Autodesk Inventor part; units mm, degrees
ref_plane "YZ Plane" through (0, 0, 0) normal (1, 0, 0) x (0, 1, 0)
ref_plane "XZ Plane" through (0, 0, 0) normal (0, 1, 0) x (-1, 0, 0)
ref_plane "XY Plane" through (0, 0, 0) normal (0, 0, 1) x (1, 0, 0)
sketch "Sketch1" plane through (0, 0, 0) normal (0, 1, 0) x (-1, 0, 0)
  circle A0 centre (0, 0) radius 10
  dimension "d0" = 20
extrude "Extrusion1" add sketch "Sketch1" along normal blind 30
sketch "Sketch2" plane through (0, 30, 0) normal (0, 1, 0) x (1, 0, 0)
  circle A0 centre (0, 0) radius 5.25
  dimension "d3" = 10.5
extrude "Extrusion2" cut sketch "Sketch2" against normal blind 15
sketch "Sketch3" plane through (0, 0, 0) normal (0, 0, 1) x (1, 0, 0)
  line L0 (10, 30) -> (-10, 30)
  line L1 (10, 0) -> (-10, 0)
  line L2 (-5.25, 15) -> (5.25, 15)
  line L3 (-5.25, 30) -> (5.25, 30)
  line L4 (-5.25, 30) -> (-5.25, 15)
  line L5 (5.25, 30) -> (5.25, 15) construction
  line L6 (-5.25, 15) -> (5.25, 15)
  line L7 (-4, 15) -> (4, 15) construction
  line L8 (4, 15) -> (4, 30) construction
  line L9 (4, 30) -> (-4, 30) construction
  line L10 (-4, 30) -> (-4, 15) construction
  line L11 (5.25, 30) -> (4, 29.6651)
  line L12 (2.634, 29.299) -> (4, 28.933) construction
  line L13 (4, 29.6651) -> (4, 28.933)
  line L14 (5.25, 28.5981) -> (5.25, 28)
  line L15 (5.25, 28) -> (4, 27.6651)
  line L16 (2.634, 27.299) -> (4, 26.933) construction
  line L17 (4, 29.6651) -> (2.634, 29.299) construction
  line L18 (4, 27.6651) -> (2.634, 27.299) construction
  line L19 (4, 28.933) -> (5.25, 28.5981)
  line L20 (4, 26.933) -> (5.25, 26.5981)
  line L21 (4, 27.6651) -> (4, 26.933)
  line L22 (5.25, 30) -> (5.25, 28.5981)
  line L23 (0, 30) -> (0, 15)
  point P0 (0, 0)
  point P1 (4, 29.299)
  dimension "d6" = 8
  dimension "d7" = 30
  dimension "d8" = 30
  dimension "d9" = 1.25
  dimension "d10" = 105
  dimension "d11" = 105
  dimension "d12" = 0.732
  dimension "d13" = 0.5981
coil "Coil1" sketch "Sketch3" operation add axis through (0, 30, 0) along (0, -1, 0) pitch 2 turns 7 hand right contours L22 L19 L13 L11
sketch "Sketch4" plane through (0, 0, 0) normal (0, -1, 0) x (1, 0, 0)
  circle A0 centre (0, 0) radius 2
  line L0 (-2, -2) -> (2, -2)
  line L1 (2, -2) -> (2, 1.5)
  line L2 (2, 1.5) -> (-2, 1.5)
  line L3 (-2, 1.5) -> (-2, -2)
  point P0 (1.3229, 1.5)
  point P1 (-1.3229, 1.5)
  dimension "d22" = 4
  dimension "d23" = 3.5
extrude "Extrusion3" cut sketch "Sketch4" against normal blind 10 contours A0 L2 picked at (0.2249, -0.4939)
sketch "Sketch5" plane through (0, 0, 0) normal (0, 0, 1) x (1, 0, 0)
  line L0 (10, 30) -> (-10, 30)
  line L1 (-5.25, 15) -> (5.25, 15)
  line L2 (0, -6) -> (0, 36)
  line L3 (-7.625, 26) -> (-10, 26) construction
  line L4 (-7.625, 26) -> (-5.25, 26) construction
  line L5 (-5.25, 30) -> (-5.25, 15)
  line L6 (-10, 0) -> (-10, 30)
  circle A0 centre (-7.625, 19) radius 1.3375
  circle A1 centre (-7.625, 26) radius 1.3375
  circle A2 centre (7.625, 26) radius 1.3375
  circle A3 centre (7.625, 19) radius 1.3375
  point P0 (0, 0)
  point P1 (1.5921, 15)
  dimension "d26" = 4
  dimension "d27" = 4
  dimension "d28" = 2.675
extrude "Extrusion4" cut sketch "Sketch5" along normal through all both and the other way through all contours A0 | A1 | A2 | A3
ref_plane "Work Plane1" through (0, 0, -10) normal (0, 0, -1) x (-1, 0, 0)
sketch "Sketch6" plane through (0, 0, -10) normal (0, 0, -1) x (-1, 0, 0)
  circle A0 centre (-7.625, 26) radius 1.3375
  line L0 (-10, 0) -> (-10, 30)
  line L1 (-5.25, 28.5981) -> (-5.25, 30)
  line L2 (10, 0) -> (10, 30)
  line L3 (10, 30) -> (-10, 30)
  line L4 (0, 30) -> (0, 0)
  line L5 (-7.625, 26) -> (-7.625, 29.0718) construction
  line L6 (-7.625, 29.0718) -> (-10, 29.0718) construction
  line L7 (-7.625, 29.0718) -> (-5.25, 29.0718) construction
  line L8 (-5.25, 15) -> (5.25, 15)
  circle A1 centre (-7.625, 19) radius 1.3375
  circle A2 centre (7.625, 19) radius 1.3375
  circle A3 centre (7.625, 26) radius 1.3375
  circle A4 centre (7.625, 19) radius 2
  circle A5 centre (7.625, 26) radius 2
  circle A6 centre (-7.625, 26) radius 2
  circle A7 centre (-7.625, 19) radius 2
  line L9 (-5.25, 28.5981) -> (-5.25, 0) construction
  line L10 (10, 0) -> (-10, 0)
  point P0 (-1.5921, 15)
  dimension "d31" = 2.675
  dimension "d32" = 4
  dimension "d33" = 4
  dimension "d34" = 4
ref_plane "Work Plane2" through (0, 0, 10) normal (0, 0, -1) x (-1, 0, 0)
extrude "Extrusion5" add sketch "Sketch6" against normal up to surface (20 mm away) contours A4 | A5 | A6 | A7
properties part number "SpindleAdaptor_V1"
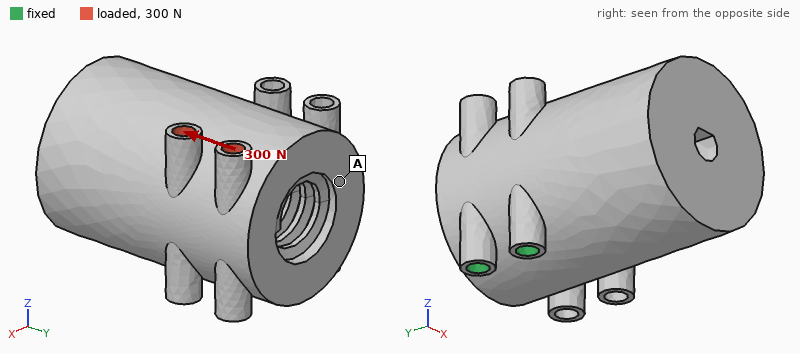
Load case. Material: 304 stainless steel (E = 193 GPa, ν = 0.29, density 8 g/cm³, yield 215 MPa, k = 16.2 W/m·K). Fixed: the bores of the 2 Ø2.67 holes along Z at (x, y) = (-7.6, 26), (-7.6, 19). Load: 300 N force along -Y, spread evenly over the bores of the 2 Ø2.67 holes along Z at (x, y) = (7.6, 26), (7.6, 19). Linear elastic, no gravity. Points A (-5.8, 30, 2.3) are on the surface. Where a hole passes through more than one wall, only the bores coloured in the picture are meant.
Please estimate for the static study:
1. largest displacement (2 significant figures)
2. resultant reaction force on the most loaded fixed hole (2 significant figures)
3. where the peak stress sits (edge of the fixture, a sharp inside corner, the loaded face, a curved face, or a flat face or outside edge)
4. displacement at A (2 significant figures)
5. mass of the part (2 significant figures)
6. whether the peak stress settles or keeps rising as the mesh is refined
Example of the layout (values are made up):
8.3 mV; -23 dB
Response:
11 µm; 830 N; edge of the fixture; 3.8 µm; 66 g; keeps rising
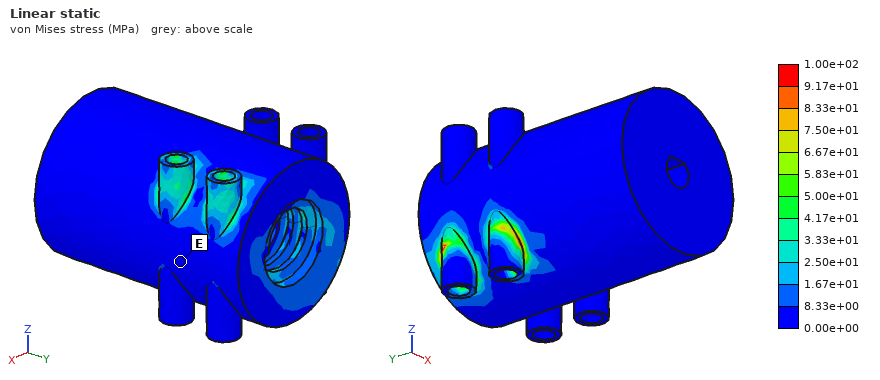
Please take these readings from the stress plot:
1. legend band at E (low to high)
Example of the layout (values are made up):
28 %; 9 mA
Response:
0.00e+00 to 8.33e+00 MPa
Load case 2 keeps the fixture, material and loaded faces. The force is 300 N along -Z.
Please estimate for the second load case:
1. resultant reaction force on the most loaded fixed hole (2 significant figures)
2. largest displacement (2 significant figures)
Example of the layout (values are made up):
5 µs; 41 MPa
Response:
160 N; 25 µm
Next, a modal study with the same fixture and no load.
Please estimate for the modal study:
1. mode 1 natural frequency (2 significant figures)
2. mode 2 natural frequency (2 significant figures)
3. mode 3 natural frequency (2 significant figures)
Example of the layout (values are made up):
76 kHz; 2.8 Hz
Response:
3100 Hz; 5000 Hz; 7200 Hz
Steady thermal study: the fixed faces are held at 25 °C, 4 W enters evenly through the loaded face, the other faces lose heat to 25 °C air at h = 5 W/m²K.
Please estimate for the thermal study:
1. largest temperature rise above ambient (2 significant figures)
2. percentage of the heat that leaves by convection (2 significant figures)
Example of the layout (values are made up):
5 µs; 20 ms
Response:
76 K; 13 %
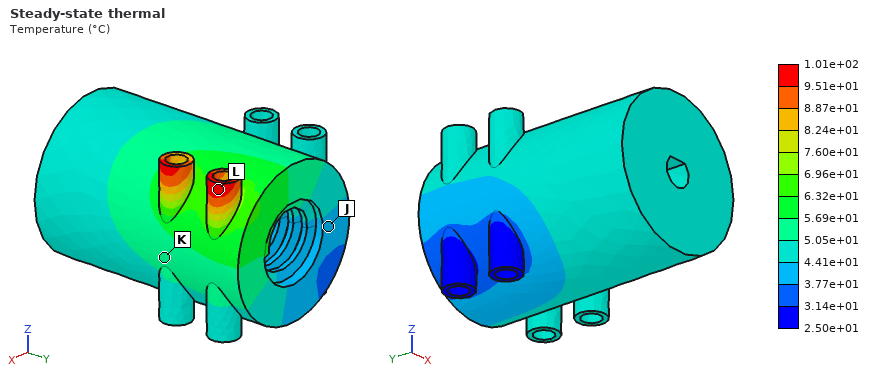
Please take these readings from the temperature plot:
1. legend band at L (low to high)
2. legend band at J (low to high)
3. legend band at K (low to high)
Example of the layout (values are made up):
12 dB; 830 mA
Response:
9.51e+01 to 1.01e+02 °C; 3.77e+01 to 4.41e+01 °C; 5.05e+01 to 5.69e+01 °C
